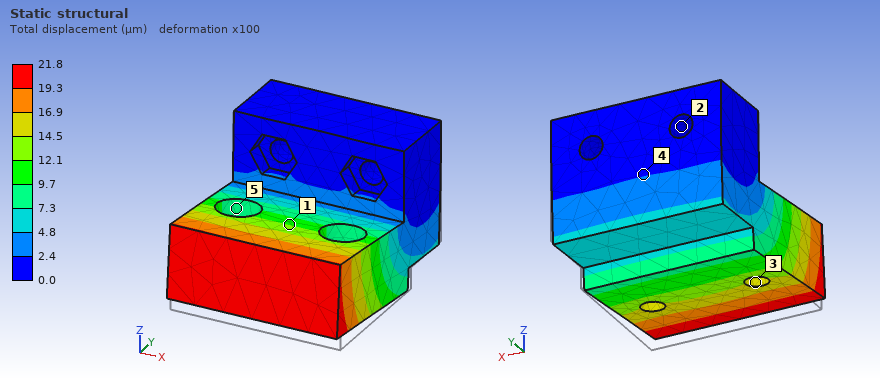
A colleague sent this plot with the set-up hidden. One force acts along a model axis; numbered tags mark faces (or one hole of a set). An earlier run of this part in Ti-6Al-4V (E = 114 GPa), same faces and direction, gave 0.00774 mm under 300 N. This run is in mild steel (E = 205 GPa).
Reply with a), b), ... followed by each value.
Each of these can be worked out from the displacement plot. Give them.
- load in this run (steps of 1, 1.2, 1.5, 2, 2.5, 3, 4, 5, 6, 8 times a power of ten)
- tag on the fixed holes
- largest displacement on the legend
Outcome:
a) 1.5 kN
b) 2
c) 21.8 µm
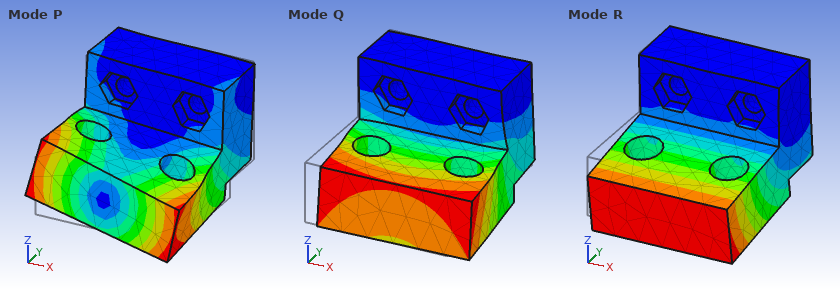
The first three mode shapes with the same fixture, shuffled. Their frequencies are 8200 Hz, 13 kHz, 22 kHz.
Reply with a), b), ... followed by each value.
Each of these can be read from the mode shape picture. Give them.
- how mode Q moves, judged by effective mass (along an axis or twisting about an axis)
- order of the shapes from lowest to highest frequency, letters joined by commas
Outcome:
a) along X
b) R, Q, P
